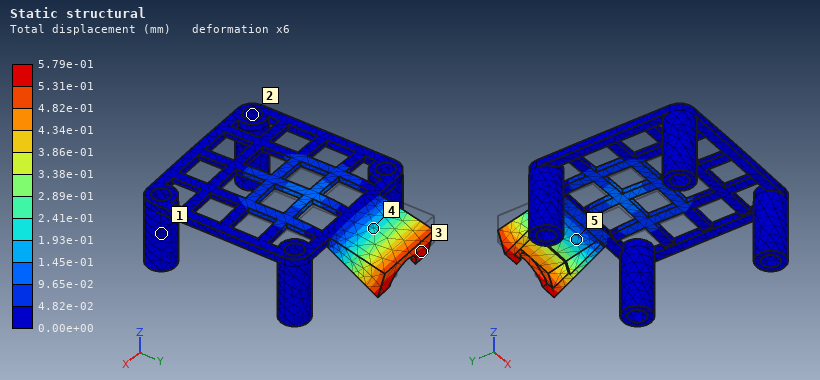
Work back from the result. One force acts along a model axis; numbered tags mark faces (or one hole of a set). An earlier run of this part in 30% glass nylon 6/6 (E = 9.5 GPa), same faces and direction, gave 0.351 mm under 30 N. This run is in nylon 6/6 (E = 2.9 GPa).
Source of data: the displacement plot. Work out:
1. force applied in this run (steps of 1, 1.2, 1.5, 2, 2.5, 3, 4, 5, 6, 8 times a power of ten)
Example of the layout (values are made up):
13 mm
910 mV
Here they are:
15 N
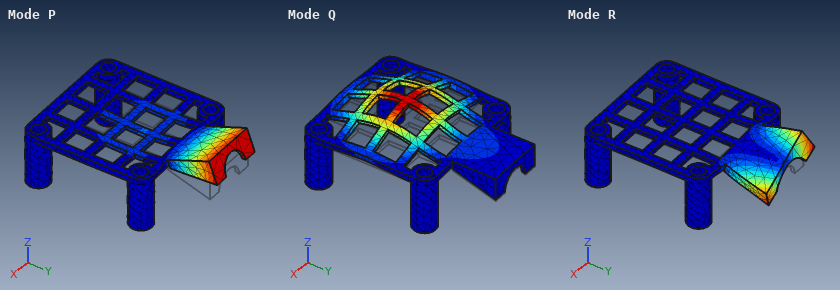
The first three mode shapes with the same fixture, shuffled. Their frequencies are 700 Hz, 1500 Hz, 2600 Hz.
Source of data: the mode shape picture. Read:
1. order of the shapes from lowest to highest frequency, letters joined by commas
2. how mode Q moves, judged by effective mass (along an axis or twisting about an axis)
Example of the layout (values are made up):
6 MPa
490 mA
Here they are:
P, Q, R
along Z
